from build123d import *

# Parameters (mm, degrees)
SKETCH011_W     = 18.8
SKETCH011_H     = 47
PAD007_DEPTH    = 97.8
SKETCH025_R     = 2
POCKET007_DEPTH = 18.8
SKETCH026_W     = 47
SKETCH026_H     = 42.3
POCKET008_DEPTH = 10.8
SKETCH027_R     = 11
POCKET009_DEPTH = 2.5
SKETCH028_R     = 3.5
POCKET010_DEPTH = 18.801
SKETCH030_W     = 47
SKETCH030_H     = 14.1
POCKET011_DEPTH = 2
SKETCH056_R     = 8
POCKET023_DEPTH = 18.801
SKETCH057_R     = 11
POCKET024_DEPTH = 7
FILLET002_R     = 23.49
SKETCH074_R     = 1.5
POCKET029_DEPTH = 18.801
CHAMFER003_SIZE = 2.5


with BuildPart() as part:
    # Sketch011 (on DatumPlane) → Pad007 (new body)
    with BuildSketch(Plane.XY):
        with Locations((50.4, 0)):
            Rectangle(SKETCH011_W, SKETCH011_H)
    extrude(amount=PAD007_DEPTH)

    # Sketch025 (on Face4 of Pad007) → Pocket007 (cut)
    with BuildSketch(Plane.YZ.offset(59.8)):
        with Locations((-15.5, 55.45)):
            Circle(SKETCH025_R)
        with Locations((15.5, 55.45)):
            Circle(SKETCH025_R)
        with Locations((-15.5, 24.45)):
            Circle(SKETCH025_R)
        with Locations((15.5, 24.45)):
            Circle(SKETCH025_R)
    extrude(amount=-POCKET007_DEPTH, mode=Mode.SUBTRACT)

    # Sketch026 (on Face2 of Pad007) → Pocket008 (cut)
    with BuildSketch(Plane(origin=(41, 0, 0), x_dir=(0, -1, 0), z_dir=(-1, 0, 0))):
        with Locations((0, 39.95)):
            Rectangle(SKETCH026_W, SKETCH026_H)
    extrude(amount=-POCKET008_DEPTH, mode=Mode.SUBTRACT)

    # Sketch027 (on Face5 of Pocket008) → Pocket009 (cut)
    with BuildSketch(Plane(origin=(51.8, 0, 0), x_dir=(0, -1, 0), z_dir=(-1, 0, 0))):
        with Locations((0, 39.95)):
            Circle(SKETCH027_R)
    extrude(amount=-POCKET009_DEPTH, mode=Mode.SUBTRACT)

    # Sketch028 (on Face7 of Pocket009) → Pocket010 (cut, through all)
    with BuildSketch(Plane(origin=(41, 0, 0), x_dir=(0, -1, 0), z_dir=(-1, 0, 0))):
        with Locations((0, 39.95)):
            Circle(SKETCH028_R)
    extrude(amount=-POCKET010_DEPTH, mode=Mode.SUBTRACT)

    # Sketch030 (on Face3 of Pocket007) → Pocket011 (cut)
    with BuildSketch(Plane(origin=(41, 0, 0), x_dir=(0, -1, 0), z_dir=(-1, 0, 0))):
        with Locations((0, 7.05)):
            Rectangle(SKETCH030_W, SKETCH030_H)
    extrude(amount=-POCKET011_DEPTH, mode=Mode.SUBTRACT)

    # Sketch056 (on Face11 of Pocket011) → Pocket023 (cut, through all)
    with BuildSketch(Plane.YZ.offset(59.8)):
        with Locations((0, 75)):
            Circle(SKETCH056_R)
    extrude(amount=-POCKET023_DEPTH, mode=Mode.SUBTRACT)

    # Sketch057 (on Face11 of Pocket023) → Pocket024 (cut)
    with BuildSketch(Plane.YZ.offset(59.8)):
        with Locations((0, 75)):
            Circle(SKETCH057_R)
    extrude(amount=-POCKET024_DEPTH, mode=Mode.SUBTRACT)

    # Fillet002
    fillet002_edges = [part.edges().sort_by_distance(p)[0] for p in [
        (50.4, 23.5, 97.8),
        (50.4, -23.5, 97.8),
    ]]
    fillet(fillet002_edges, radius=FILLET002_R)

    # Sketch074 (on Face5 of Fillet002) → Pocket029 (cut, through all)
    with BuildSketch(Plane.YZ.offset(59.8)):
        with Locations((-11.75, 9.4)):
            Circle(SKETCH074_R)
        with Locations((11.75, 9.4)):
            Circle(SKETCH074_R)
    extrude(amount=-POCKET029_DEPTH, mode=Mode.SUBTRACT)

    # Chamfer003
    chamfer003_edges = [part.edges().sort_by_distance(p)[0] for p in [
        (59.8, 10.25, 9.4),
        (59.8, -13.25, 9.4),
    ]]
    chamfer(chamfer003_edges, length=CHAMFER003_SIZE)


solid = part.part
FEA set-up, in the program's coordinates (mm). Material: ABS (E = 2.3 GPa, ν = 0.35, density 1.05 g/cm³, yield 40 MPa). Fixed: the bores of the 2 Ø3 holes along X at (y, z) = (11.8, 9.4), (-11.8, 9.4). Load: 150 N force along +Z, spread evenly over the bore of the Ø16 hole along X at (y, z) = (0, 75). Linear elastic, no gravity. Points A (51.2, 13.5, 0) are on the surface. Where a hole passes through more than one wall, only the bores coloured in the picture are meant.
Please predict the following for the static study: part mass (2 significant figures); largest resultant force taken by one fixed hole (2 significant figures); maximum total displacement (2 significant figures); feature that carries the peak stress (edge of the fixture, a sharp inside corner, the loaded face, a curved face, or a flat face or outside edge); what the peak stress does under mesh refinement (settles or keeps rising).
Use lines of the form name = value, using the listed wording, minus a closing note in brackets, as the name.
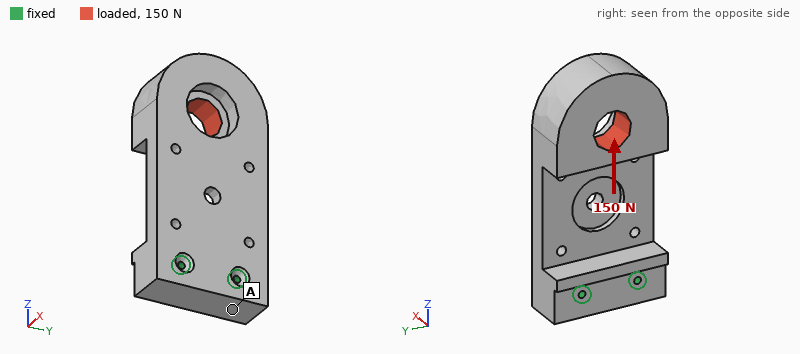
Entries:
part mass = 55 g
largest resultant force taken by one fixed hole = 75 N
maximum total displacement = 1.1 mm
feature that carries the peak stress = a sharp inside corner
what the peak stress does under mesh refinement = keeps rising
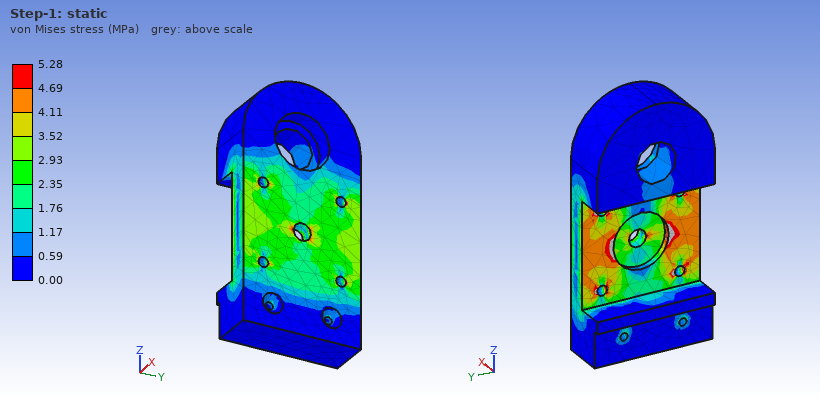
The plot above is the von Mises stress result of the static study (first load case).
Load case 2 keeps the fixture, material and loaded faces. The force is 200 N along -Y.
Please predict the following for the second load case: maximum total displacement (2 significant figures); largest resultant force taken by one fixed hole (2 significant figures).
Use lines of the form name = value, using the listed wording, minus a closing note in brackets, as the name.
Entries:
maximum total displacement = 0.58 mm
largest resultant force taken by one fixed hole = 530 N
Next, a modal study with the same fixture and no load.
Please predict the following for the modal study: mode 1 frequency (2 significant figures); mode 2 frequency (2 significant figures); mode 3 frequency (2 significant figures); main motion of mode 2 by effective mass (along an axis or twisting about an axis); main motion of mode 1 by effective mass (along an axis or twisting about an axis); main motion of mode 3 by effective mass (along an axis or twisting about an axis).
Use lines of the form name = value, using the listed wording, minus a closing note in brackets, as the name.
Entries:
mode 1 frequency = 200 Hz
mode 2 frequency = 650 Hz
mode 3 frequency = 970 Hz
main motion of mode 2 by effective mass = along Y
main motion of mode 1 by effective mass = along X
main motion of mode 3 by effective mass = along Y
